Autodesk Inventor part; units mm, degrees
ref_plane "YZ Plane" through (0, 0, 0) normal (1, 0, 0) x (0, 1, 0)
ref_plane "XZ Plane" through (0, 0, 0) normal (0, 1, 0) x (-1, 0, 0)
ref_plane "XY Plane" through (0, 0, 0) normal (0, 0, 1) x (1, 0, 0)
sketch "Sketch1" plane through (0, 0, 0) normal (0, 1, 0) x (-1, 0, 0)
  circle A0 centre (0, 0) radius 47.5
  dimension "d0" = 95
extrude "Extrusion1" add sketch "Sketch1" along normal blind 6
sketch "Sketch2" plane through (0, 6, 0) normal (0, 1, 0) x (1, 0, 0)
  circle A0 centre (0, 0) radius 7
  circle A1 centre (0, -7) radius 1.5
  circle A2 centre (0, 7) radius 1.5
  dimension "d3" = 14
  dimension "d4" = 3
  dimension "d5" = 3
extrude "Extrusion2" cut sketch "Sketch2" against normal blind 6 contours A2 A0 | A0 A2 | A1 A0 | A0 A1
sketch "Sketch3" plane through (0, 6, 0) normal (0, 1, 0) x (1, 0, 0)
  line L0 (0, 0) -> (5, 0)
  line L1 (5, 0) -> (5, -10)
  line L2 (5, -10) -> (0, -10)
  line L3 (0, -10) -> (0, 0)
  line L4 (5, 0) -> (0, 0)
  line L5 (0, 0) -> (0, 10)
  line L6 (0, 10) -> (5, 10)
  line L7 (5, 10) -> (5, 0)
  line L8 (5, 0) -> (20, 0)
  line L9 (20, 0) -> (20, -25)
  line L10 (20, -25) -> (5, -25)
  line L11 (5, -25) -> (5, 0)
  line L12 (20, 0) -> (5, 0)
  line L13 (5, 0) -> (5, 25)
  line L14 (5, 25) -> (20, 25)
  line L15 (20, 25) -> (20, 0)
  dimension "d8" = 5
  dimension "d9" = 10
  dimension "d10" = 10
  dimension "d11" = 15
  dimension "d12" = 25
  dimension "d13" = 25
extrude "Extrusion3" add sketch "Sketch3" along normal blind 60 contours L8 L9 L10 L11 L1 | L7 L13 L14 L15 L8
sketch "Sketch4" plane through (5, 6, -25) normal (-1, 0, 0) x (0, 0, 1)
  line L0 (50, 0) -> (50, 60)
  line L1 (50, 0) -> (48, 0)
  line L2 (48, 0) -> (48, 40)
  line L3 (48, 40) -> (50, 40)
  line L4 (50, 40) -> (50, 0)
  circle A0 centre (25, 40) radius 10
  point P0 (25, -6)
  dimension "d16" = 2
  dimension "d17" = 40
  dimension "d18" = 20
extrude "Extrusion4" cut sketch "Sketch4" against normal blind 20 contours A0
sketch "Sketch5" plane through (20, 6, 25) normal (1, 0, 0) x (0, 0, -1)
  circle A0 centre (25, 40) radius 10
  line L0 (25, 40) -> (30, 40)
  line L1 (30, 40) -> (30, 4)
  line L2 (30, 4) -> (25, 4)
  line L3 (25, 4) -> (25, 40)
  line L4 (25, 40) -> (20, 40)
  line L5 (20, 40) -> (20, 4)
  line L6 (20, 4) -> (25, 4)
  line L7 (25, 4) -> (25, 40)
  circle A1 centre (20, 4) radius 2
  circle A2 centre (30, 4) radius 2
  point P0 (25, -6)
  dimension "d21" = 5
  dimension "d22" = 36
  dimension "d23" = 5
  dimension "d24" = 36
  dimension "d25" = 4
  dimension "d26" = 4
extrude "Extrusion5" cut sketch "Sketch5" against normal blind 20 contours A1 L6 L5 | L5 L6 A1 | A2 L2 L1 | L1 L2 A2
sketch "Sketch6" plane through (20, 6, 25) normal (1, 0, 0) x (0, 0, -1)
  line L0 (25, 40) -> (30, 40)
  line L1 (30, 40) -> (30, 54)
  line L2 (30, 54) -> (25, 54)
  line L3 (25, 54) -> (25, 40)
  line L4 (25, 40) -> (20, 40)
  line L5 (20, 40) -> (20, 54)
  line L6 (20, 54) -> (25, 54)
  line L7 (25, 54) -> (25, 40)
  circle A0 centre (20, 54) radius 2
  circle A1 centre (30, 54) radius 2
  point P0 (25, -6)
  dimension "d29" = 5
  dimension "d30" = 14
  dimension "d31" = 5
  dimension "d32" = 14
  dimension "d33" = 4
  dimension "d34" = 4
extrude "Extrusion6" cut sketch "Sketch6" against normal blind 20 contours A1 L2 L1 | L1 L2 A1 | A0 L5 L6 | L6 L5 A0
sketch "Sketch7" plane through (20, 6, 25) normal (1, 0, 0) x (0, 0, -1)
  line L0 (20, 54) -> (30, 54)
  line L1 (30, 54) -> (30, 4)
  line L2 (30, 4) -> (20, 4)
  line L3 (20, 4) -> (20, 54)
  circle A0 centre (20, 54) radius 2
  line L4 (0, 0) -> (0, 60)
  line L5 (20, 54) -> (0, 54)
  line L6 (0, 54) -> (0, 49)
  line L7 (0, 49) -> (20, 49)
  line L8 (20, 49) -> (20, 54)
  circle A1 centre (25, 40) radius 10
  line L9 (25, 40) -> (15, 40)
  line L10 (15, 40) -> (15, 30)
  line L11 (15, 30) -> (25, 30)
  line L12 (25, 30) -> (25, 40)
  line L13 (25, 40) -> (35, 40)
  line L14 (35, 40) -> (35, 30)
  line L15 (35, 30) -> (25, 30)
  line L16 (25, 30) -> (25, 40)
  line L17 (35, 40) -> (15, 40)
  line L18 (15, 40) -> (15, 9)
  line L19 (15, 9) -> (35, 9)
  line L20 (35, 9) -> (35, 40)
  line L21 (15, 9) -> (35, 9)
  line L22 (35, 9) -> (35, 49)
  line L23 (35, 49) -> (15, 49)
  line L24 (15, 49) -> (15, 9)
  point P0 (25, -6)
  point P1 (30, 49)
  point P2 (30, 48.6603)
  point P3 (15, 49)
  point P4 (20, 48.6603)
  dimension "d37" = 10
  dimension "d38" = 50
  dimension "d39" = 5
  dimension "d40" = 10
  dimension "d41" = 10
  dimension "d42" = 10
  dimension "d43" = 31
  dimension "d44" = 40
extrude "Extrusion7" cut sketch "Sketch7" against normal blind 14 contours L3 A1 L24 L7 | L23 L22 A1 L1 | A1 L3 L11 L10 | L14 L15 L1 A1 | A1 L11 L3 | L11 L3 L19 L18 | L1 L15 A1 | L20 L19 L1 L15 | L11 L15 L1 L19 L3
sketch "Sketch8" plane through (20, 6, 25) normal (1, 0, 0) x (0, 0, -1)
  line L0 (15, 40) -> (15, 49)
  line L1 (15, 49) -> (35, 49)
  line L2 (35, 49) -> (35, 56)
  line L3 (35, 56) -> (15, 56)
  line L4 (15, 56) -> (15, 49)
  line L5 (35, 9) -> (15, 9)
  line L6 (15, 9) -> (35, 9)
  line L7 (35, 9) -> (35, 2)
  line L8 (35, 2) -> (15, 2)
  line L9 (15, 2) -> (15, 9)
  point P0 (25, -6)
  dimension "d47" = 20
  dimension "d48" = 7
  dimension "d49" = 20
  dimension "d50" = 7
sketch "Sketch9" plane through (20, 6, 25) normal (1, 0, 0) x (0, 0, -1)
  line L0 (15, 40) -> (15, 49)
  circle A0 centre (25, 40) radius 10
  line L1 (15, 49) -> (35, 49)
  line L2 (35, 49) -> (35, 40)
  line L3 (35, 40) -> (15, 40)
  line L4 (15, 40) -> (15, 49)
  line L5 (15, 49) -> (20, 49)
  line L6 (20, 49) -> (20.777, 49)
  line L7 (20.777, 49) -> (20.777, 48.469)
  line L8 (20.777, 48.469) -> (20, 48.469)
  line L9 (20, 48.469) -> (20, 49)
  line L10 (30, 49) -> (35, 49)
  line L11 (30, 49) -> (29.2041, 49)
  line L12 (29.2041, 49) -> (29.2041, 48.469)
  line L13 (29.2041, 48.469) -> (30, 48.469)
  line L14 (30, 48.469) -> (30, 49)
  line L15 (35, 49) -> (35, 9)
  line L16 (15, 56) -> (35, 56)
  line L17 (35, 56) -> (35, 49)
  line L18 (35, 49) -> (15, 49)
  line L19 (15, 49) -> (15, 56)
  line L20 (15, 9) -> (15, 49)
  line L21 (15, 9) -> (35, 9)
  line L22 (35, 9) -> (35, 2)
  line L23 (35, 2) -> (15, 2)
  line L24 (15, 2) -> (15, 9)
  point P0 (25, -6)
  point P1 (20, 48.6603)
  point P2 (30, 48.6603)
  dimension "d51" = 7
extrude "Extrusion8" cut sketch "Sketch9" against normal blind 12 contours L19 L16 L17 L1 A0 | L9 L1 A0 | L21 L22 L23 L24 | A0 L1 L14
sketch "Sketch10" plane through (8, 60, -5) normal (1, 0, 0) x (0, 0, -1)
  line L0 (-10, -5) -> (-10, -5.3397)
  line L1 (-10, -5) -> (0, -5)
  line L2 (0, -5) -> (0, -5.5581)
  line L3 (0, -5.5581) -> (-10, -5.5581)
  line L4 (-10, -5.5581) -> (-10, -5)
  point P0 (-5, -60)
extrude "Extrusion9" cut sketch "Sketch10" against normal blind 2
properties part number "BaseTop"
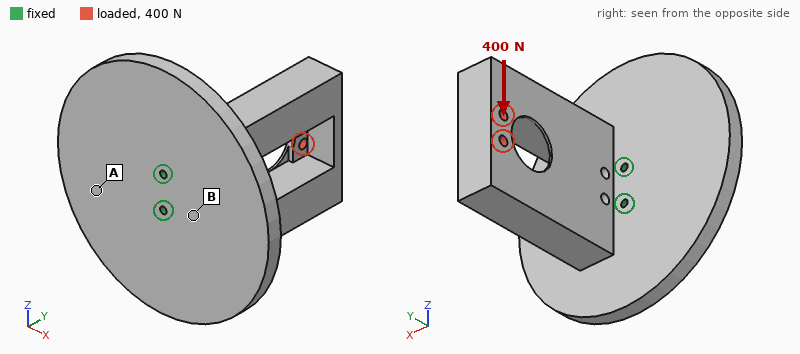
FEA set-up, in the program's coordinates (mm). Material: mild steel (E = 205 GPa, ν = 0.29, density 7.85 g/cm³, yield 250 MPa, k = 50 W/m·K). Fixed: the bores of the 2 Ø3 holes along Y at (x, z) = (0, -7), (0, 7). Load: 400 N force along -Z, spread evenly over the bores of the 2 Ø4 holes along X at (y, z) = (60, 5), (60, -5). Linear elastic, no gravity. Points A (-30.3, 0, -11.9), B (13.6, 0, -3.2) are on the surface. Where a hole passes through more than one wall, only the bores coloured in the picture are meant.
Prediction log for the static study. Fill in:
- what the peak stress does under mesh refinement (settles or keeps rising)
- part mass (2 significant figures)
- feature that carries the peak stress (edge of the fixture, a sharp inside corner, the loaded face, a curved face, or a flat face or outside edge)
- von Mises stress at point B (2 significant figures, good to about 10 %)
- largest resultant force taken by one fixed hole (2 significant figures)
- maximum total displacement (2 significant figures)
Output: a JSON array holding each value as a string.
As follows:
["keeps rising", "570 g", "edge of the fixture", "9.6 MPa", "1.1 kN", "29 µm"]
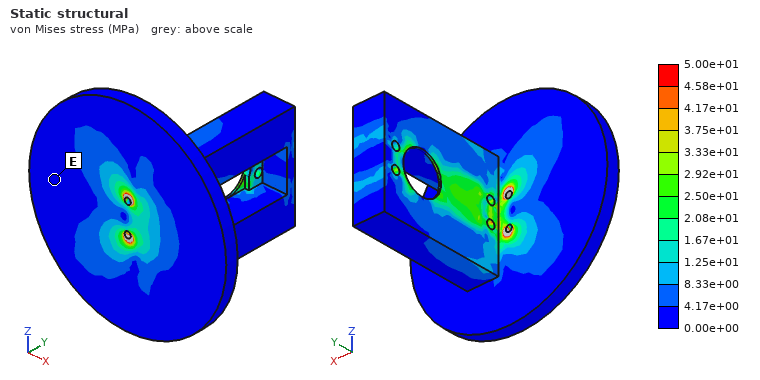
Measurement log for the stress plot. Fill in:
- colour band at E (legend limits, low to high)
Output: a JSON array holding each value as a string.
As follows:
["0.00e+00 to 4.17e+00 MPa"]
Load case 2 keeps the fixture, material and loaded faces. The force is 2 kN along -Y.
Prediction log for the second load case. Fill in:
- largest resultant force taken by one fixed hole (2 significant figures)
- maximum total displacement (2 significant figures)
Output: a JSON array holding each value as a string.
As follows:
["1.0 kN", "22 µm"]
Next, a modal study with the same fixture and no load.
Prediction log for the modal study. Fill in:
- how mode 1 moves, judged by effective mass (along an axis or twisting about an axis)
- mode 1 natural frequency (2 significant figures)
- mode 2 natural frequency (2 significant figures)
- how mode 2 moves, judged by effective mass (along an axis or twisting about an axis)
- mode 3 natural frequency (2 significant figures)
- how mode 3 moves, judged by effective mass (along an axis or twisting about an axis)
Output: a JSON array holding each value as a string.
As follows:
["along X", "950 Hz", "1700 Hz", "along Z", "2400 Hz", "along Y"]
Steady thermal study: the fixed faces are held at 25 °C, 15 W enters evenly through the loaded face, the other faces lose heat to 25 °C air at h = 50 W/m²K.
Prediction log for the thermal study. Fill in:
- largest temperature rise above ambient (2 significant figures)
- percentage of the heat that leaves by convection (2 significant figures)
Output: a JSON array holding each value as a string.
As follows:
["53 K", "69 %"]
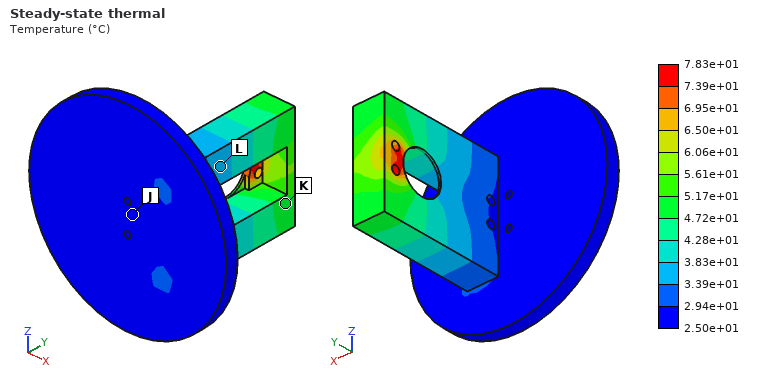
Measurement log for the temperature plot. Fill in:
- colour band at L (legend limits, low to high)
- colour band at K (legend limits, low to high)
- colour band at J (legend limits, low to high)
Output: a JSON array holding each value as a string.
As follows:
["3.39e+01 to 3.83e+01 °C", "4.72e+01 to 5.17e+01 °C", "2.50e+01 to 2.94e+01 °C"]
